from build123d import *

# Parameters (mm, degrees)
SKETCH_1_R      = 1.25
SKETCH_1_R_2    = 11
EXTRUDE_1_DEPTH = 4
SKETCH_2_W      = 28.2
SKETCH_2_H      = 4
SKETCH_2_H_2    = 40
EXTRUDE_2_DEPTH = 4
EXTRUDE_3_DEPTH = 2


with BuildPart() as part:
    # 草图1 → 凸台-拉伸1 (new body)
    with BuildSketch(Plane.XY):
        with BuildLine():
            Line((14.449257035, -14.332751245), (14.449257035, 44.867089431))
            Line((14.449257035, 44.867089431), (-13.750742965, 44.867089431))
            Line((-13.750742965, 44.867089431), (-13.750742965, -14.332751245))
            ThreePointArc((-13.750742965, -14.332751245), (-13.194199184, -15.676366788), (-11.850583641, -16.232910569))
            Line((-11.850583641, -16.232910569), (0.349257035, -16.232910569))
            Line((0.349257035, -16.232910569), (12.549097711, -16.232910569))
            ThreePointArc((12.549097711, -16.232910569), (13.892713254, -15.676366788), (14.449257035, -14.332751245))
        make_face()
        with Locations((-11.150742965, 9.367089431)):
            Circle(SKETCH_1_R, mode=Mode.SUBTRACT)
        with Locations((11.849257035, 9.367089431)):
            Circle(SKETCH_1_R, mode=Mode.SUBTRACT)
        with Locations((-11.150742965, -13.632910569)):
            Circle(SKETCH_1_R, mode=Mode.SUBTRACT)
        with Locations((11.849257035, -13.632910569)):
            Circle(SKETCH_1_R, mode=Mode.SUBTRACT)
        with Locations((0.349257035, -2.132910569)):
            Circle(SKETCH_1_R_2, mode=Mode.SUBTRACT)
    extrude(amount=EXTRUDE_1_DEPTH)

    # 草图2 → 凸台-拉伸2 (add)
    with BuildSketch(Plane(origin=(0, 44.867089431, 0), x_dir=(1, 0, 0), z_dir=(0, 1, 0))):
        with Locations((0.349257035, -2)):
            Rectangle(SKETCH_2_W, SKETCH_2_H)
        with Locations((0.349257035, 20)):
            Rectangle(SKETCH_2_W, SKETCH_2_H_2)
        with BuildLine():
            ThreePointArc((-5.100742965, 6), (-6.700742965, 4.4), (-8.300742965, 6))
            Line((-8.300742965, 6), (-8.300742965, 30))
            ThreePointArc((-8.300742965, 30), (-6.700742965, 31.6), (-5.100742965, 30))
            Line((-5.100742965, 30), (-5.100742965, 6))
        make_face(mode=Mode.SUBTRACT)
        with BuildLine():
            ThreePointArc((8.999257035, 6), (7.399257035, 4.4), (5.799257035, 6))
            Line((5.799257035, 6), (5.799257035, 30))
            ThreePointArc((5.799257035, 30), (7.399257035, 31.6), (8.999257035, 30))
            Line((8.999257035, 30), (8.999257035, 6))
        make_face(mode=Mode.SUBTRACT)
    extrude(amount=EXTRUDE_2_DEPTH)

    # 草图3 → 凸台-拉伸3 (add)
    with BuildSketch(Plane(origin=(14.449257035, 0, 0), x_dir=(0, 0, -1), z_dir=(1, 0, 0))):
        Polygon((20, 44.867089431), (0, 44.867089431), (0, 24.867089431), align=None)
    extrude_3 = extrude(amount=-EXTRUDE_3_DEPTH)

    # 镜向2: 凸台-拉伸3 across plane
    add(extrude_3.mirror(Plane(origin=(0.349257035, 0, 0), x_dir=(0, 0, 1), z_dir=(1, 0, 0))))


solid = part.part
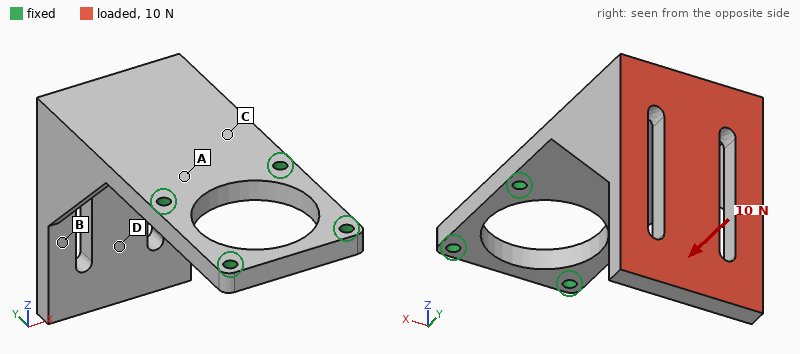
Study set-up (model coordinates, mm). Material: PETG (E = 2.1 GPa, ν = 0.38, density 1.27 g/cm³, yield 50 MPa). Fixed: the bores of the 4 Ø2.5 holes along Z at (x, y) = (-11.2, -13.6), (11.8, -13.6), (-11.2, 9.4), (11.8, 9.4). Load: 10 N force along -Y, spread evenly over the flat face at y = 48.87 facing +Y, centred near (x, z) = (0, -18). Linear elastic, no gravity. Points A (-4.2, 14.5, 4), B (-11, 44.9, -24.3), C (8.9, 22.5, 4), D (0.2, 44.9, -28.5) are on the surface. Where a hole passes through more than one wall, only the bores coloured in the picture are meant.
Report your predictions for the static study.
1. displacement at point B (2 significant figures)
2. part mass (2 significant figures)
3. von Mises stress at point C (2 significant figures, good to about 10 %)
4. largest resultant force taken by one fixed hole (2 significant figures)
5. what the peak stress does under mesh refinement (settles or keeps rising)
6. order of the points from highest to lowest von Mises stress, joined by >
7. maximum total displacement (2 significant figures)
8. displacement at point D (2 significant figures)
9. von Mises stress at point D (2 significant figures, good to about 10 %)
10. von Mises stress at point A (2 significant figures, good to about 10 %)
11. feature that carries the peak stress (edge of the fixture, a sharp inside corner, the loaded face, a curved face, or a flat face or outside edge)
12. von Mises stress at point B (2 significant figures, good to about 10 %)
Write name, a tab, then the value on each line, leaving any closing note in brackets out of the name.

displacement at point B	0.60 mm
part mass	13 g
von Mises stress at point C	2.6 MPa
largest resultant force taken by one fixed hole	5.1 N
what the peak stress does under mesh refinement	keeps rising
order of the points from highest to lowest von Mises stress, joined by >	C > A > B > D
maximum total displacement	0.90 mm
displacement at point D	0.67 mm
von Mises stress at point D	0.42 MPa
von Mises stress at point A	2.2 MPa
feature that carries the peak stress	edge of the fixture
von Mises stress at point B	0.85 MPa
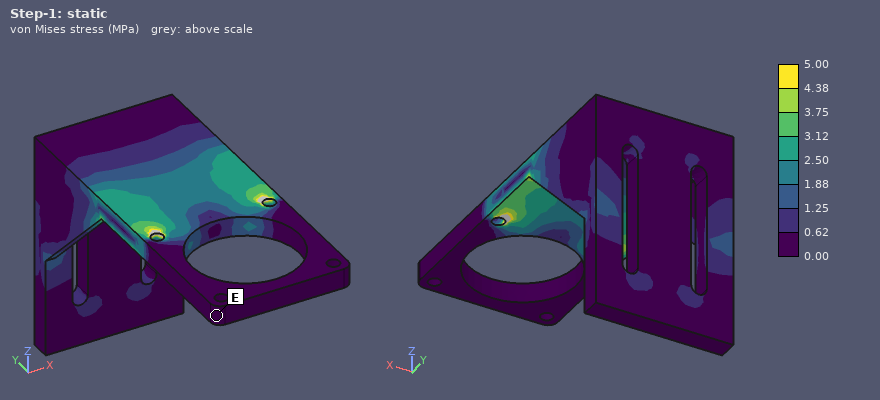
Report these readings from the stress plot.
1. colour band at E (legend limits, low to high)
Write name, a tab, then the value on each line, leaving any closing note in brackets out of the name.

colour band at E	0.00 to 0.62 MPa
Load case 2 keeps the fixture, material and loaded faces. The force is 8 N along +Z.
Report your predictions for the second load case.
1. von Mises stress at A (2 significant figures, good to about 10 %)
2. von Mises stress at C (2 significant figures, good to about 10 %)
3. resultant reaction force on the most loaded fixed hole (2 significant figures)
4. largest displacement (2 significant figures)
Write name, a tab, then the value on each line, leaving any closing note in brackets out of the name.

von Mises stress at A	2.9 MPa
von Mises stress at C	2.8 MPa
resultant reaction force on the most loaded fixed hole	4.6 N
largest displacement	0.98 mm
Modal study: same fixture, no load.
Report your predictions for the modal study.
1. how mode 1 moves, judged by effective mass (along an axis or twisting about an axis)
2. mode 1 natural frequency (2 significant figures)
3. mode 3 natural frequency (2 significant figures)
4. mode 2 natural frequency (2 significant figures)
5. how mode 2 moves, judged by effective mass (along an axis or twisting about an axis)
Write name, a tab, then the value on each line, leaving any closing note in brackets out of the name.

how mode 1 moves, judged by effective mass	along Z
mode 1 natural frequency	190 Hz
mode 3 natural frequency	830 Hz
mode 2 natural frequency	360 Hz
how mode 2 moves, judged by effective mass	along X
